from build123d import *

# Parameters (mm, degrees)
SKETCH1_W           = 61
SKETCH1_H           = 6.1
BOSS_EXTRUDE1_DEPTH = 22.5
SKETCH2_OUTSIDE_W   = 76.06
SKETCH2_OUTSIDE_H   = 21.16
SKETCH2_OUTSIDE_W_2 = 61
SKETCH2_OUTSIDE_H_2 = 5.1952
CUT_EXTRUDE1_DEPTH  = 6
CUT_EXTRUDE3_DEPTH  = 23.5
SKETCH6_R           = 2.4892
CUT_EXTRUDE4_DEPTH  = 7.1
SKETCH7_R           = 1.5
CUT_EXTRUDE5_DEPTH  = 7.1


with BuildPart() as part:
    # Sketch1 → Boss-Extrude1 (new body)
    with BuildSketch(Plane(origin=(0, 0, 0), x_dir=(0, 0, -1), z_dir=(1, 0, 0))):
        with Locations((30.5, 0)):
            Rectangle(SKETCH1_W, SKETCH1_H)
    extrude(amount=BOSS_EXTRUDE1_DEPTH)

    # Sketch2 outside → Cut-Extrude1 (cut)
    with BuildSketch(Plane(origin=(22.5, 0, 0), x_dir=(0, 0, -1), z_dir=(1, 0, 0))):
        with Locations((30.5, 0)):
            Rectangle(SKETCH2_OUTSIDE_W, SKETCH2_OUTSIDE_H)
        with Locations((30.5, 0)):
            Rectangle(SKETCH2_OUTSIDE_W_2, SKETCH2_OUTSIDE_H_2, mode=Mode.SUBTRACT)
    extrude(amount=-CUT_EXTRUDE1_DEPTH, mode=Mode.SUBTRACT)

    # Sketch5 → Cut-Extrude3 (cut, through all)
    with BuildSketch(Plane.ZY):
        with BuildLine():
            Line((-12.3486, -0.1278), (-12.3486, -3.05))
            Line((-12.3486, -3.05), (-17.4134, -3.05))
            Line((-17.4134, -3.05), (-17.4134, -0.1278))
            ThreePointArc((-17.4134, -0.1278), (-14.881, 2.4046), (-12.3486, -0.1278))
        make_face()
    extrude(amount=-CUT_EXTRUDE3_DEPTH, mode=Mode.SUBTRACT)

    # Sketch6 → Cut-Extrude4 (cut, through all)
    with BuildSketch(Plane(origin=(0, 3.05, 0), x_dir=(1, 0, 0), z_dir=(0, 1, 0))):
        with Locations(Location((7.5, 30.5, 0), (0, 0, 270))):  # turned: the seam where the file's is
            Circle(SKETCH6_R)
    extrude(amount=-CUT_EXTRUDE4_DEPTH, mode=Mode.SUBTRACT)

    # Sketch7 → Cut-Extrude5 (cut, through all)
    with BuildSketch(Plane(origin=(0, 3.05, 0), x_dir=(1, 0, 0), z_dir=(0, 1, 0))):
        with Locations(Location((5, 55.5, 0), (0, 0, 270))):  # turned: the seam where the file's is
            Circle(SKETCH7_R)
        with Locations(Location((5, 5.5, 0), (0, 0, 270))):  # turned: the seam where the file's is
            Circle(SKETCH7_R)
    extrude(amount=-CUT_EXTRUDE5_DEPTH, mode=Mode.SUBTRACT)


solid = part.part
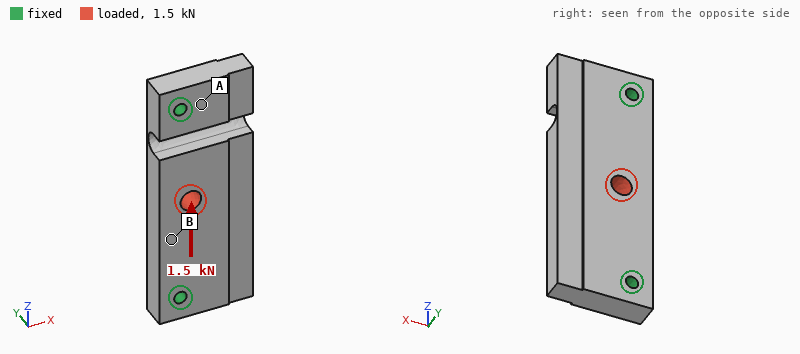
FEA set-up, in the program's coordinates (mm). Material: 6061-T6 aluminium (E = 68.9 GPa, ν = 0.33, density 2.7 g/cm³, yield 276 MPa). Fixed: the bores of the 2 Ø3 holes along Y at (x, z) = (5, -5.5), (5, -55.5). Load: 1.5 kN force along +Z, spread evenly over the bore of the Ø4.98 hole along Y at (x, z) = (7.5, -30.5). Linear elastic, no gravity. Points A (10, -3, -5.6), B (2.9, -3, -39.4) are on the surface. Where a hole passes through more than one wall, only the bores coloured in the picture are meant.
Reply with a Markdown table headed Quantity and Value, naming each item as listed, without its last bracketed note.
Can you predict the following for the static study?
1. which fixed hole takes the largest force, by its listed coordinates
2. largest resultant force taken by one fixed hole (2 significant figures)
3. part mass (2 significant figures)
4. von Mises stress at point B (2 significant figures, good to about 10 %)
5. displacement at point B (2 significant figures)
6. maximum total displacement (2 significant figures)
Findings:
| Quantity | Value |
|---|---|
| which fixed hole takes the largest force, by its listed coordinates | (5, -55.5) |
| largest resultant force taken by one fixed hole | 1.2 kN |
| part mass | 20 g |
| von Mises stress at point B | 18 MPa |
| displacement at point B | 4.3 µm |
| maximum total displacement | 8.7 µm |
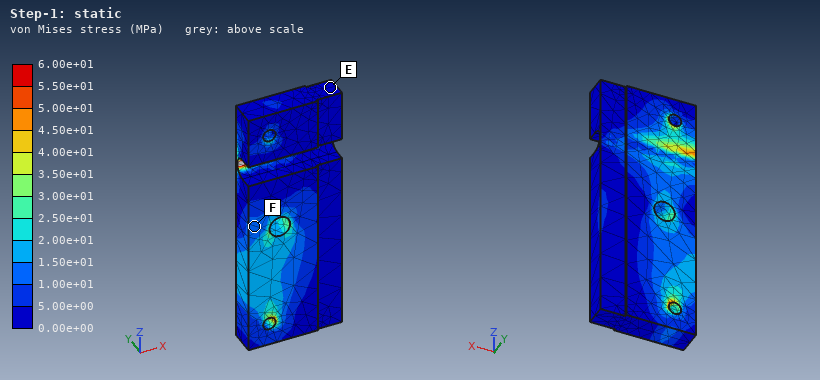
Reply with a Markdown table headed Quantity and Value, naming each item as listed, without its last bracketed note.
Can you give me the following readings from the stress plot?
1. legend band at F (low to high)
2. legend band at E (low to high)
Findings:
| Quantity | Value |
|---|---|
| legend band at F | 1.00e+01 to 1.50e+01 MPa |
| legend band at E | 0.00e+00 to 5.00e+00 MPa |
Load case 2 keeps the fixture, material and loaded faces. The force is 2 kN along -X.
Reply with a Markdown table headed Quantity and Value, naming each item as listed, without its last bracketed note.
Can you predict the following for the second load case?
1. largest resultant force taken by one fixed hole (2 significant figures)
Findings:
| Quantity | Value |
|---|---|
| largest resultant force taken by one fixed hole | 1.1 kN |
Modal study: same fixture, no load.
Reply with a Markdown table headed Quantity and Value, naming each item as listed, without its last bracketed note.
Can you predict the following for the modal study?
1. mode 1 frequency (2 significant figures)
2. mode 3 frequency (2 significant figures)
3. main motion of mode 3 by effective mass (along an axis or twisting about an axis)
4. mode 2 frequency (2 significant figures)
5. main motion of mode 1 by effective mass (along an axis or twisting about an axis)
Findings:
| Quantity | Value |
|---|---|
| mode 1 frequency | 6600 Hz |
| mode 3 frequency | 14 kHz |
| main motion of mode 3 by effective mass | along X |
| mode 2 frequency | 9900 Hz |
| main motion of mode 1 by effective mass | along Y |
